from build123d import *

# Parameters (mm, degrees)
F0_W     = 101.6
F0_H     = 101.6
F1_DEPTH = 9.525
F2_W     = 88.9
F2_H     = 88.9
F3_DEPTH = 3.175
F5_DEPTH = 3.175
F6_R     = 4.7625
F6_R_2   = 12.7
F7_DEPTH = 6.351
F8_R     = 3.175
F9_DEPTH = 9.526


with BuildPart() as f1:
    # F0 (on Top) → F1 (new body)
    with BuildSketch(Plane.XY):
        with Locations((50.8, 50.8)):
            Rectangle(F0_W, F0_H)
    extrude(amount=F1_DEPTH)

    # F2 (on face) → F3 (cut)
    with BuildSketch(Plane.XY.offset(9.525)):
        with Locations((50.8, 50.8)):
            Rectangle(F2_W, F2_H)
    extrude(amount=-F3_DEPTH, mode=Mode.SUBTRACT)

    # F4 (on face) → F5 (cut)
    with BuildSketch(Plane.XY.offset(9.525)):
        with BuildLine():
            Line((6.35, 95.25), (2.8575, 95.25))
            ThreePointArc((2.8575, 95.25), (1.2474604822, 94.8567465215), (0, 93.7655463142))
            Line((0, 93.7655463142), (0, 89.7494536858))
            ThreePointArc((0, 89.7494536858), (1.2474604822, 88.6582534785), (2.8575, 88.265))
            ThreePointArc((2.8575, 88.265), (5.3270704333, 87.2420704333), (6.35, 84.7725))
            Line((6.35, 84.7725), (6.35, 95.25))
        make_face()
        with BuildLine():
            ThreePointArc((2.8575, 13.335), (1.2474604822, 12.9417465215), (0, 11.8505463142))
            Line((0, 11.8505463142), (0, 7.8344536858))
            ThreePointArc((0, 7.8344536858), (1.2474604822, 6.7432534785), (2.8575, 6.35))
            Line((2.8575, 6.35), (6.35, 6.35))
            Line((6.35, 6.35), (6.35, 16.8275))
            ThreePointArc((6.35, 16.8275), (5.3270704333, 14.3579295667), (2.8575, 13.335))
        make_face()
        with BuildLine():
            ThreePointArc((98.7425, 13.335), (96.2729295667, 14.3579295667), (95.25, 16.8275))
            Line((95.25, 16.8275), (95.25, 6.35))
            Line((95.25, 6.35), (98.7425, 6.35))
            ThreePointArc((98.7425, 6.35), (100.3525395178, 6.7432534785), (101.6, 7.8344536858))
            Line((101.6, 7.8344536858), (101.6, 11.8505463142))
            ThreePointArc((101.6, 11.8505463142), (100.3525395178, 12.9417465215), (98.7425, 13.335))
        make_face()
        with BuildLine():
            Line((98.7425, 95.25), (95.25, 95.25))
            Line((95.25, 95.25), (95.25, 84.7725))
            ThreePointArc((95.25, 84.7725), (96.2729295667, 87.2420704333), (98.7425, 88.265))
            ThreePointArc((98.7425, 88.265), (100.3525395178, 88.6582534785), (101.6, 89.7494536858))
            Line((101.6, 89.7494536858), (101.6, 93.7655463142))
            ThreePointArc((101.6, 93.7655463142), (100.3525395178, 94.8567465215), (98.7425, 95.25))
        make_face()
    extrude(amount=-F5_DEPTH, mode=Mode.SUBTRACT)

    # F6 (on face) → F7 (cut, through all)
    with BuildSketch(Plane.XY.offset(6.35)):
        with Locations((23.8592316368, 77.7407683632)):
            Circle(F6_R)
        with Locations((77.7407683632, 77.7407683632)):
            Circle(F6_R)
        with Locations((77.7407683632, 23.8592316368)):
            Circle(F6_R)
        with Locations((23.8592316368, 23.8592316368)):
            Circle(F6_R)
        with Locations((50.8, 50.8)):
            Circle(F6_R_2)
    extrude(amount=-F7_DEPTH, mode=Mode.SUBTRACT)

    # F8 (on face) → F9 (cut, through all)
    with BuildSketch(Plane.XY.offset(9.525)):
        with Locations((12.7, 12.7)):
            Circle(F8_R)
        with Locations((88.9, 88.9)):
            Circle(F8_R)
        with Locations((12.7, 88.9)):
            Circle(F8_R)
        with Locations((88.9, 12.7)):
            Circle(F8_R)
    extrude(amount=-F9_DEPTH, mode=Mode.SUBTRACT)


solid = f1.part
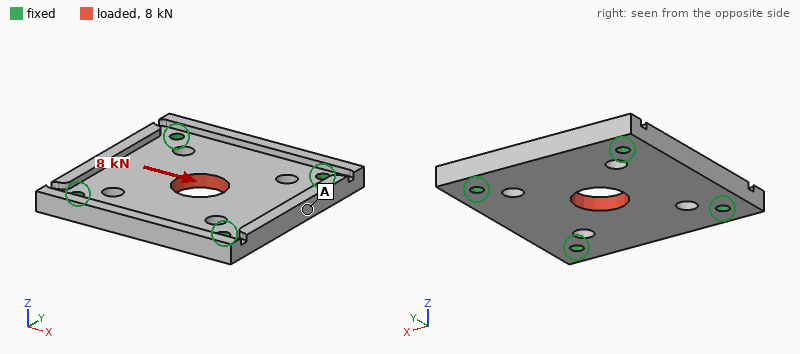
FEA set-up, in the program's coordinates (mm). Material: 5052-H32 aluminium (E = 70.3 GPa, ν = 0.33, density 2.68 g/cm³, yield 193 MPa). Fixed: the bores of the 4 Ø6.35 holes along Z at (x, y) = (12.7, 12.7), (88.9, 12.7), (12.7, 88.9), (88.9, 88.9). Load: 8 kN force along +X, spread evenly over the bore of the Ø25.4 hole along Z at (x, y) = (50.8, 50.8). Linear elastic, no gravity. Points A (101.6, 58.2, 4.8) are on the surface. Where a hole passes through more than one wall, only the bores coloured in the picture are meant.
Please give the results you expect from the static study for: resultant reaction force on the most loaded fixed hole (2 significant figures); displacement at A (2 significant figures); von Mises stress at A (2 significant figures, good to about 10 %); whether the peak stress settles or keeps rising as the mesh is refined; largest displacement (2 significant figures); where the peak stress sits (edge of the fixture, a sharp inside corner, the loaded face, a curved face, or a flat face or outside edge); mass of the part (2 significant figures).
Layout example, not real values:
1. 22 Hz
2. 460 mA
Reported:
1. 2.1 kN
2. 10 µm
3. 11 MPa
4. keeps rising
5. 14 µm
6. edge of the fixture
7. 180 g
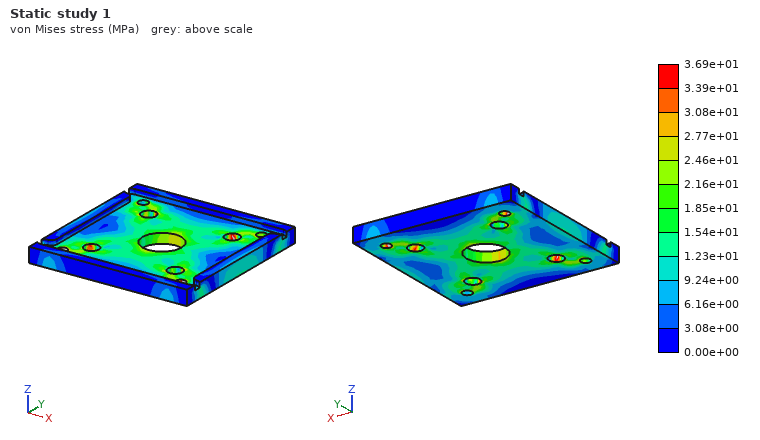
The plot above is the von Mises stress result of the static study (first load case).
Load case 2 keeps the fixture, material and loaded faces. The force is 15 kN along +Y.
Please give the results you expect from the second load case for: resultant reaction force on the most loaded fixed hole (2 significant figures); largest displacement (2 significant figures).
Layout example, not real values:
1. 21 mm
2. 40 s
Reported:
1. 4.0 kN
2. 26 µm
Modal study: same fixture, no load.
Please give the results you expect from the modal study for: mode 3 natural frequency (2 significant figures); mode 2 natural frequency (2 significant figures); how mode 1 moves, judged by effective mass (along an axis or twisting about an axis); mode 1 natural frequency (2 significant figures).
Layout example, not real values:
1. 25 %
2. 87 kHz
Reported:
1. 6300 Hz
2. 6200 Hz
3. along Z
4. 4200 Hz
